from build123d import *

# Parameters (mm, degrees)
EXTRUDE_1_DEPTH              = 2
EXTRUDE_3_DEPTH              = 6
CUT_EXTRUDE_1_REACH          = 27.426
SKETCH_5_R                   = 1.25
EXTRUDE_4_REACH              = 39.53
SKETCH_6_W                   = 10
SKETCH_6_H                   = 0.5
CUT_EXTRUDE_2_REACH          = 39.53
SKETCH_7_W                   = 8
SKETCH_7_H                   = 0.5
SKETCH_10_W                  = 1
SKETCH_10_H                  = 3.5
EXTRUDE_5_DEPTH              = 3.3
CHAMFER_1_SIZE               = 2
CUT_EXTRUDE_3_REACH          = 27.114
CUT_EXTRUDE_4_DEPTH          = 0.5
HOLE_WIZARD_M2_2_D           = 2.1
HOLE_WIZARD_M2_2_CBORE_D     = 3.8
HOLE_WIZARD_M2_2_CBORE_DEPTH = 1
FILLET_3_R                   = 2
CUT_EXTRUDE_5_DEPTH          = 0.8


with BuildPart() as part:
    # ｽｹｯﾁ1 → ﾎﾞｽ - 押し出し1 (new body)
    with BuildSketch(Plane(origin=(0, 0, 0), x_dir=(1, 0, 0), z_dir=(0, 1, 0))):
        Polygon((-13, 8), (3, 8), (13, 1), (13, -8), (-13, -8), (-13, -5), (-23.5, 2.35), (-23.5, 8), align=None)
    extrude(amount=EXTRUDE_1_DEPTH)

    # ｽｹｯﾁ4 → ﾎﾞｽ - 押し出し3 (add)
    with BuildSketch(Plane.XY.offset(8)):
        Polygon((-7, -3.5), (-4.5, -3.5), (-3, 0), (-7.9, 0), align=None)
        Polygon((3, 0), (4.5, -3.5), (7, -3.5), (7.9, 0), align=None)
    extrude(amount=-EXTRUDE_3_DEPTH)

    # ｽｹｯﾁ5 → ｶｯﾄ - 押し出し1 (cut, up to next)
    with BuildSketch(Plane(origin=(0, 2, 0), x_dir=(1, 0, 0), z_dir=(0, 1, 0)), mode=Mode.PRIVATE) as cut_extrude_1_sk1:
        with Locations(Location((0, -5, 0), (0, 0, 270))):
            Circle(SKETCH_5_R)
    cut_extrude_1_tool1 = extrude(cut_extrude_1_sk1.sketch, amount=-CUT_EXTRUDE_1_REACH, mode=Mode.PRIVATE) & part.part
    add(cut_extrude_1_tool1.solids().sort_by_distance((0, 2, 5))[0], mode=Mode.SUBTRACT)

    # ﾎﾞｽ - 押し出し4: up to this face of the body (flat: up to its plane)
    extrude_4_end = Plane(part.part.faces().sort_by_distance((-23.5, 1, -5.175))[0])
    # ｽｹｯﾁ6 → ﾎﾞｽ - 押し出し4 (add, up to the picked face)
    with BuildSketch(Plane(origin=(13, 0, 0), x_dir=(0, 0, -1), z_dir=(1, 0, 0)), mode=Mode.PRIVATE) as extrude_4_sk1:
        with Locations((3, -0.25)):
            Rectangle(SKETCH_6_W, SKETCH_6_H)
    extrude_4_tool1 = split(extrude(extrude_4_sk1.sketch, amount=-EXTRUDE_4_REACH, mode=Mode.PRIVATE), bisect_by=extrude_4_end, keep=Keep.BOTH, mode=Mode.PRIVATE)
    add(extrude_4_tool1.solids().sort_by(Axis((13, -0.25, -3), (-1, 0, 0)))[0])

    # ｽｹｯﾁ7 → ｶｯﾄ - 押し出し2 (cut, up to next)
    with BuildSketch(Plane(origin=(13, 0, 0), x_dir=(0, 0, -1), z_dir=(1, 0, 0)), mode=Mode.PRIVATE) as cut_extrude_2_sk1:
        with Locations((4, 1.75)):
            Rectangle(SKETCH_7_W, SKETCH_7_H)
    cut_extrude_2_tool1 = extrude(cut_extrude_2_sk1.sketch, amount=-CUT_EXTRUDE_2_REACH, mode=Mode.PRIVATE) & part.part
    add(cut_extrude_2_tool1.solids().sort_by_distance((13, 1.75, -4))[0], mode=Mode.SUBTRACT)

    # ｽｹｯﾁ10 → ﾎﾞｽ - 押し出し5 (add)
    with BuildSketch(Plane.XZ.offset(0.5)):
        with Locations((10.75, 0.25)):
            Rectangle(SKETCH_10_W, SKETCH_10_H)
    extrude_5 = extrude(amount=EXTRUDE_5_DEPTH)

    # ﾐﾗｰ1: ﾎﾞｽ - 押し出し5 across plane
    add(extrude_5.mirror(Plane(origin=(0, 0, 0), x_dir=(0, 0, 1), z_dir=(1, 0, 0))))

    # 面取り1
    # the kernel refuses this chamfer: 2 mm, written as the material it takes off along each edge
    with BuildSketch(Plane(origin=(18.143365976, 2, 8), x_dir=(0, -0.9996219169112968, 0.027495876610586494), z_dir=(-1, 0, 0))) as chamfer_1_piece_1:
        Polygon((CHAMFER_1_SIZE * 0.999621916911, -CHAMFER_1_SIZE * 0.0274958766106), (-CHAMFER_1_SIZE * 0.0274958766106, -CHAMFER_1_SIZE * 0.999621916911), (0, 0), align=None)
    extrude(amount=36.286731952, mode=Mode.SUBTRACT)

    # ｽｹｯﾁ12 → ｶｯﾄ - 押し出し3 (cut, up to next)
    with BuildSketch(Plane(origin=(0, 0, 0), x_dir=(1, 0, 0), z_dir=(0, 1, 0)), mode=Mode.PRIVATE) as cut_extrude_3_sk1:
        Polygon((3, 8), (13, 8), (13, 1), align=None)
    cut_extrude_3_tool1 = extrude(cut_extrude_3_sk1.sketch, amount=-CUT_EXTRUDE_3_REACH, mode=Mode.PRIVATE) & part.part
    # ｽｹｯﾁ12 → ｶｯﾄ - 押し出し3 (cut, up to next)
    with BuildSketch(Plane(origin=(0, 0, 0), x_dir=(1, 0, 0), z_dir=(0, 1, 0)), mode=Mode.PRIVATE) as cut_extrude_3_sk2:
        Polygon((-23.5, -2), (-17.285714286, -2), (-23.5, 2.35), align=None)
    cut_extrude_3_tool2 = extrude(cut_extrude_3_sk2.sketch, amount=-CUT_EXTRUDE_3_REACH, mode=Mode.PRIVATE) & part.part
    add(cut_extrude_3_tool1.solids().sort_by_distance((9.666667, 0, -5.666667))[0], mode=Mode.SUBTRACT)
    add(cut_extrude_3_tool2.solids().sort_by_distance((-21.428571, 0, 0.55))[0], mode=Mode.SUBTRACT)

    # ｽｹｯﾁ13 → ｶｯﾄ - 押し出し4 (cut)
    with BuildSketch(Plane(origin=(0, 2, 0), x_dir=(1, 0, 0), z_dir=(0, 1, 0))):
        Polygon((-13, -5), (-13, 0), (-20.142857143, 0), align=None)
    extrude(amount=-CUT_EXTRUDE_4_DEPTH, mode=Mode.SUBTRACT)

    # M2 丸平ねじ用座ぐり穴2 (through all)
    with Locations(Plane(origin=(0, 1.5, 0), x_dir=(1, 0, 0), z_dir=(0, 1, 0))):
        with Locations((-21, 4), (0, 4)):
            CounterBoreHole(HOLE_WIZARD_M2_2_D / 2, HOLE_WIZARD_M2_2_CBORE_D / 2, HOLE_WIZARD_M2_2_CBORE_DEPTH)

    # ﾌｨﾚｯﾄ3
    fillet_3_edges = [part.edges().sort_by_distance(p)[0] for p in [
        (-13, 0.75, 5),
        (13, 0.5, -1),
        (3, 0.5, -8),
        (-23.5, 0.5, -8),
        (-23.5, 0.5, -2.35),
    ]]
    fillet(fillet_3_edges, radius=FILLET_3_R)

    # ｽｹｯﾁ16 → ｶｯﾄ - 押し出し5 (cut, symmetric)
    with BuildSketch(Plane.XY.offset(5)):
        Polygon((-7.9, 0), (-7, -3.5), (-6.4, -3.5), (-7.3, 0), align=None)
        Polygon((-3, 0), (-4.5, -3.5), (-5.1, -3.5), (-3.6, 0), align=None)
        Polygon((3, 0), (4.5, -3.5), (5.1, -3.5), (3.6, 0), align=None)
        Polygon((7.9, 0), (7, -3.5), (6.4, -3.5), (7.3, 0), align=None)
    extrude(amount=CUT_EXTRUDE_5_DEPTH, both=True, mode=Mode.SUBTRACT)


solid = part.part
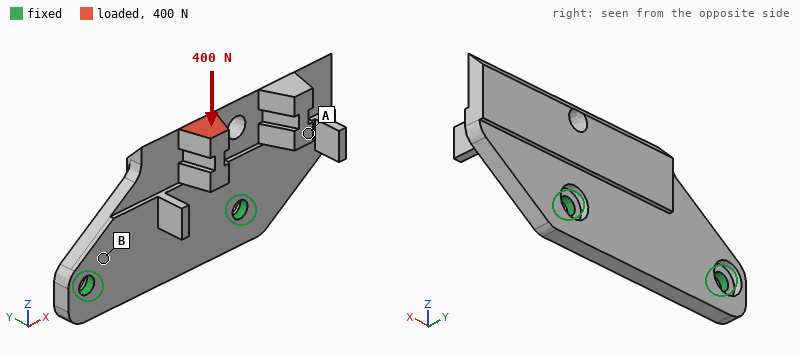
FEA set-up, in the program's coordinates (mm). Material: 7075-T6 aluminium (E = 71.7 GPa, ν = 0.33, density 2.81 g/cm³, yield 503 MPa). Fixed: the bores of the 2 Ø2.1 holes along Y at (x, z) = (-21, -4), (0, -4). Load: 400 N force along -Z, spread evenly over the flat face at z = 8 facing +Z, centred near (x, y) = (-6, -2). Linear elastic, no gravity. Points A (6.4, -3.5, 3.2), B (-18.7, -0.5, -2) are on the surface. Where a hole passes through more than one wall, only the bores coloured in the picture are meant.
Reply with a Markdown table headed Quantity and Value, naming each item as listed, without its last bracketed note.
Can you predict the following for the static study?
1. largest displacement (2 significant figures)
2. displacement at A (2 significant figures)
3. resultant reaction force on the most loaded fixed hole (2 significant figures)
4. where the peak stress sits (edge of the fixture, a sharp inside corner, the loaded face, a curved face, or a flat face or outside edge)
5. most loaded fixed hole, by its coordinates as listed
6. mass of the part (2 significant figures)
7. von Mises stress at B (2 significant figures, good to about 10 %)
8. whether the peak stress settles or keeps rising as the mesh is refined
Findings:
| Quantity | Value |
|---|---|
| largest displacement | 95 µm |
| displacement at A | 36 µm |
| resultant reaction force on the most loaded fixed hole | 300 N |
| where the peak stress sits | edge of the fixture |
| most loaded fixed hole, by its coordinates as listed | (0, -4) |
| mass of the part | 3.0 g |
| von Mises stress at B | 57 MPa |
| whether the peak stress settles or keeps rising as the mesh is refined | keeps rising |
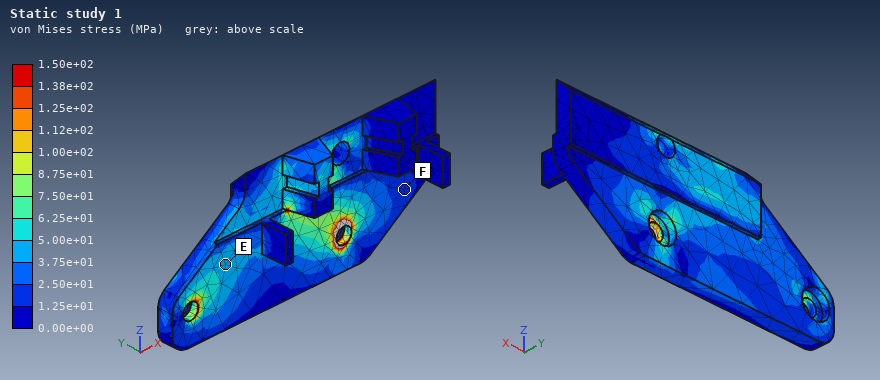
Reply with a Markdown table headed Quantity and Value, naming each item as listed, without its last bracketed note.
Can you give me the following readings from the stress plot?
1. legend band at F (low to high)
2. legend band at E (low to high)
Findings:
| Quantity | Value |
|---|---|
| legend band at F | 1.25e+01 to 2.50e+01 MPa |
| legend band at E | 3.75e+01 to 5.00e+01 MPa |
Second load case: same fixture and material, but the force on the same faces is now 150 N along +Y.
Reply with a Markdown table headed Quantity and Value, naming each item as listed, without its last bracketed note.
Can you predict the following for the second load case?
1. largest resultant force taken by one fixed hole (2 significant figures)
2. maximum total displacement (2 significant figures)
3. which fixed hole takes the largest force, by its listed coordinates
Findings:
| Quantity | Value |
|---|---|
| largest resultant force taken by one fixed hole | 140 N |
| maximum total displacement | 0.20 mm |
| which fixed hole takes the largest force, by its listed coordinates | (0, -4) |
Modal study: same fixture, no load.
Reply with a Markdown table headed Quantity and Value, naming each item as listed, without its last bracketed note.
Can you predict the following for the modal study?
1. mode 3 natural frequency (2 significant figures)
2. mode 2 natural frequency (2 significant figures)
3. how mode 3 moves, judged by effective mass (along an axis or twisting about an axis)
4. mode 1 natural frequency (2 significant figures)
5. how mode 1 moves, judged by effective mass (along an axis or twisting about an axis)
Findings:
| Quantity | Value |
|---|---|
| mode 3 natural frequency | 18 kHz |
| mode 2 natural frequency | 7800 Hz |
| how mode 3 moves, judged by effective mass | along Y |
| mode 1 natural frequency | 5200 Hz |
| how mode 1 moves, judged by effective mass | along Y |
